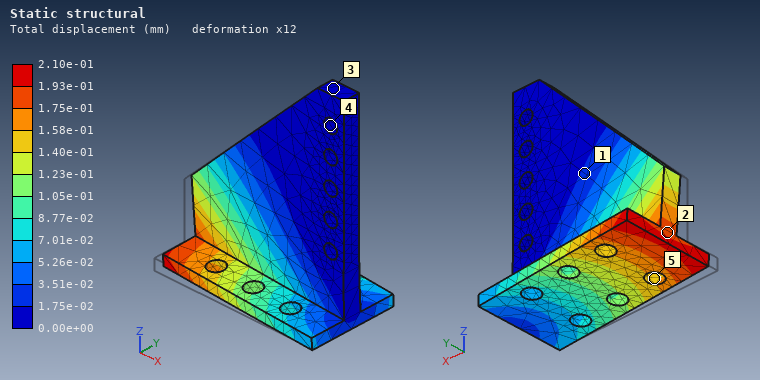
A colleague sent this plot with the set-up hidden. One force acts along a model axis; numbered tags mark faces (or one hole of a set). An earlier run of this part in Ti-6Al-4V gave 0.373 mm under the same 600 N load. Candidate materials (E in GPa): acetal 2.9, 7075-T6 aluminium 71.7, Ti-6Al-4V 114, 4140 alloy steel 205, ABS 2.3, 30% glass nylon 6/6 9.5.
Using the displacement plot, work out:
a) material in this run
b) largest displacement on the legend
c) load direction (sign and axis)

4140 alloy steel
2.10e-01 mm
+Y
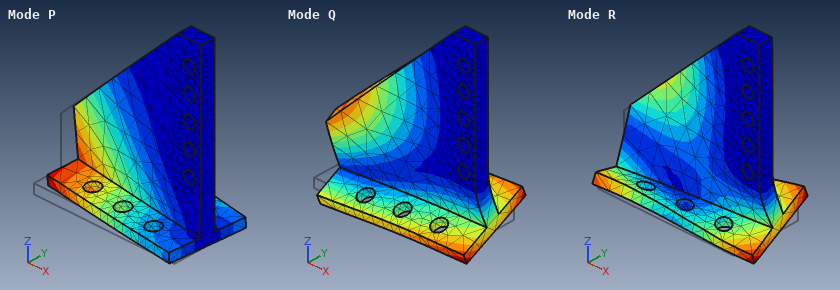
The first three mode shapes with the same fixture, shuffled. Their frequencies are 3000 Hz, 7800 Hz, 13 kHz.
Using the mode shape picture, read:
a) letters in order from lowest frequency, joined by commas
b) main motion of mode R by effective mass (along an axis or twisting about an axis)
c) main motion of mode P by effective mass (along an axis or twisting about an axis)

P, Q, R
along Y
along Y
